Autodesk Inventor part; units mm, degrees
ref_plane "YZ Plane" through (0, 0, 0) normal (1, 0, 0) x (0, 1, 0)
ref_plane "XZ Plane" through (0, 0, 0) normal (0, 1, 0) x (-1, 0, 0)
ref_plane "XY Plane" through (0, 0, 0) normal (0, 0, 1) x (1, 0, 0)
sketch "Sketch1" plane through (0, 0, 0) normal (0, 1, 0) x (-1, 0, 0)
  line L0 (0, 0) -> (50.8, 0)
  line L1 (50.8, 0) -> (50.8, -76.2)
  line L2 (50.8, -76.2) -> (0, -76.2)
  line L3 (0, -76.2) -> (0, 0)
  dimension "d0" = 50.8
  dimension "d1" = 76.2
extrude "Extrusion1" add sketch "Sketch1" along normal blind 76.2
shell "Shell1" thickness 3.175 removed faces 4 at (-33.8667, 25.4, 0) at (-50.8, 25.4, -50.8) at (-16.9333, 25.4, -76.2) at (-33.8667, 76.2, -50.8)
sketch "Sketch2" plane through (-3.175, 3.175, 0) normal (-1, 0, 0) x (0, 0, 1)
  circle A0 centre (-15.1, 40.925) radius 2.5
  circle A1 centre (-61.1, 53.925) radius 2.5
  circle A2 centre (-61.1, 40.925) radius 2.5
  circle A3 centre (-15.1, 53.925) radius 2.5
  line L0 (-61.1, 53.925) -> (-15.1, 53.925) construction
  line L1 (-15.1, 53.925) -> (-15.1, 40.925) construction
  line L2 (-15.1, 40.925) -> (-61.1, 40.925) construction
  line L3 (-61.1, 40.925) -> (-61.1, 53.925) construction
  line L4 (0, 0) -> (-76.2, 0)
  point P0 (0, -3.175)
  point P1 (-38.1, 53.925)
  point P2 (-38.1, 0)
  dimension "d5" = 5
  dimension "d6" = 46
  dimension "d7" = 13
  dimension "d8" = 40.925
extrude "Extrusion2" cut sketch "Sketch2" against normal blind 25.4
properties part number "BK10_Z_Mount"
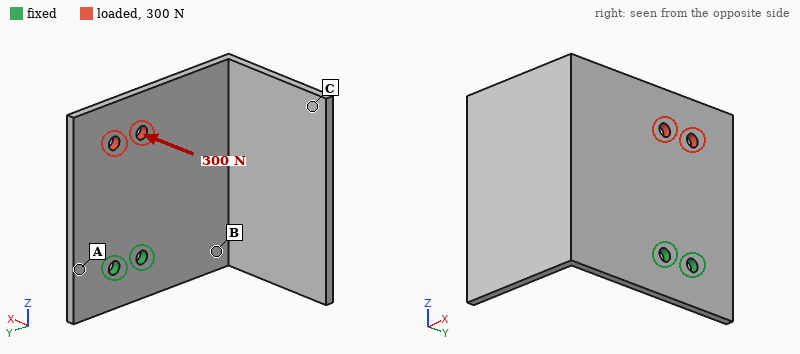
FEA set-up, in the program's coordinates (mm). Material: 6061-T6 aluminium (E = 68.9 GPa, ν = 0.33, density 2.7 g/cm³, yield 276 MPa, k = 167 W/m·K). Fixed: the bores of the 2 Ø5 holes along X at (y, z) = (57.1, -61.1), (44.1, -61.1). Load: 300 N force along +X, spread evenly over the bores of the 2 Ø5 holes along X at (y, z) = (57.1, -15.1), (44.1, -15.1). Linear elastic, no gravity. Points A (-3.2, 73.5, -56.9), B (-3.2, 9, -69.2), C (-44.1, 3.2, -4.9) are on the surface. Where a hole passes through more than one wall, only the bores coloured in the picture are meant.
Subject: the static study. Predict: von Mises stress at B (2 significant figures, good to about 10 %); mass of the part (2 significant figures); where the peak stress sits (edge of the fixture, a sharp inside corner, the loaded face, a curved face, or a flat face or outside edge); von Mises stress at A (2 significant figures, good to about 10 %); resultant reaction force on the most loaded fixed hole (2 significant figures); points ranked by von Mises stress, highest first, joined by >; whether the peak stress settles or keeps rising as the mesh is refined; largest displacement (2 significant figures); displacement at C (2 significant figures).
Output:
38 MPa
80 g
edge of the fixture
69 MPa
150 N
A > B > C
keeps rising
1.2 mm
1.0 mm
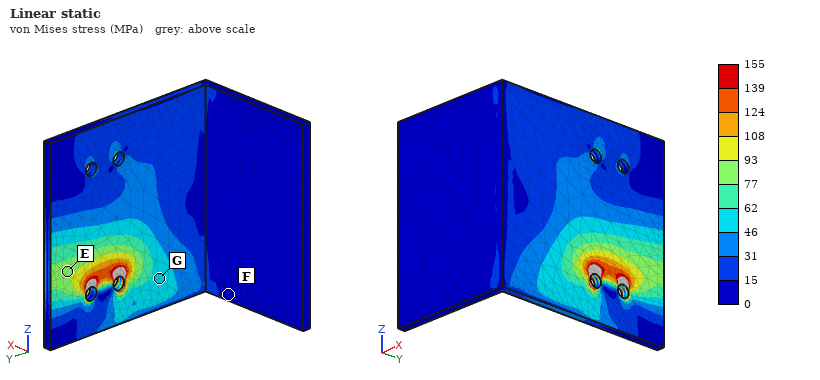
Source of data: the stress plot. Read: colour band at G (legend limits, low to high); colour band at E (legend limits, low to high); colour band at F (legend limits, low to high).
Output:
46 to 62 MPa
77 to 93 MPa
0 to 15 MPa
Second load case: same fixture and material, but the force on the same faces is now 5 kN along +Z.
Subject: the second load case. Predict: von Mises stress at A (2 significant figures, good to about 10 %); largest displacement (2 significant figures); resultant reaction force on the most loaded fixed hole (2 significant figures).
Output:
9.5 MPa
33 µm
2.5 kN
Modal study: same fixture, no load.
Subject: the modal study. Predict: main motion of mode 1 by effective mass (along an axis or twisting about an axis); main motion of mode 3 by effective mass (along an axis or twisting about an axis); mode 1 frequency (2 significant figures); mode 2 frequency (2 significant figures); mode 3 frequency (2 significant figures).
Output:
along X
along X
310 Hz
460 Hz
990 Hz
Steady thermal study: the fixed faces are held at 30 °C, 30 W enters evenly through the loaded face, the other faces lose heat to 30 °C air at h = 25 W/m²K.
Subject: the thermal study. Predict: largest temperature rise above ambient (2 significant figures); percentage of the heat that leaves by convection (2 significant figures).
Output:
45 K
28 %
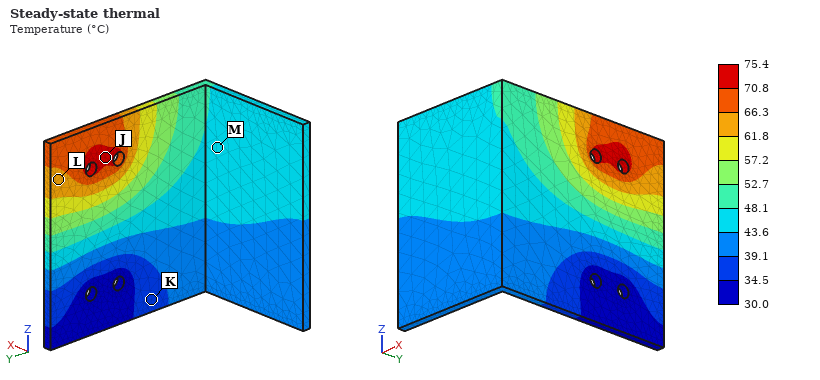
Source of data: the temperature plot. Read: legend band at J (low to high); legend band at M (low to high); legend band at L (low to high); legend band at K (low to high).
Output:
70.8 to 75.4 °C
43.6 to 48.1 °C
61.8 to 66.3 °C
34.5 to 39.1 °C
